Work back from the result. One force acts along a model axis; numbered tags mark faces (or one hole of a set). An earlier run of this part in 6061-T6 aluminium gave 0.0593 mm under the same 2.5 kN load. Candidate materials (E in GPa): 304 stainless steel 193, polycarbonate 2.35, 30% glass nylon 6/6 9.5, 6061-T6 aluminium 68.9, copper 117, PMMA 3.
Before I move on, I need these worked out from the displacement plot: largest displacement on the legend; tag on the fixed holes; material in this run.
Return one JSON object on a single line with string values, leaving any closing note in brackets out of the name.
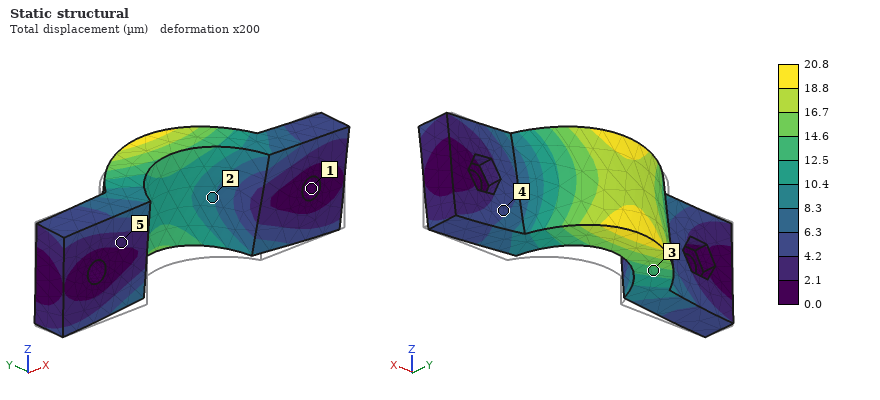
{"largest displacement on the legend": "20.8 µm", "tag on the fixed holes": "1", "material in this run": "304 stainless steel"}
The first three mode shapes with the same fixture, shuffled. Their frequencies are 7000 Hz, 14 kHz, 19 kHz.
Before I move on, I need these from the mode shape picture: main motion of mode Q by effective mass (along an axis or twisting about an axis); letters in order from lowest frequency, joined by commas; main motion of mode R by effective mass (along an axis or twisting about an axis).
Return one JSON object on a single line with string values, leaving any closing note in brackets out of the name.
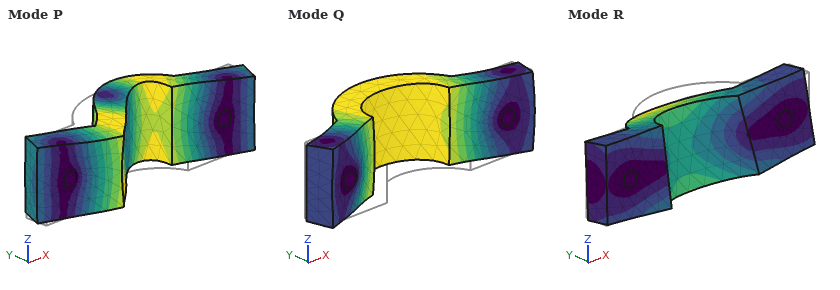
{"main motion of mode Q by effective mass": "along Y", "letters in order from lowest frequency, joined by commas": "R, Q, P", "main motion of mode R by effective mass": "along Z"}
